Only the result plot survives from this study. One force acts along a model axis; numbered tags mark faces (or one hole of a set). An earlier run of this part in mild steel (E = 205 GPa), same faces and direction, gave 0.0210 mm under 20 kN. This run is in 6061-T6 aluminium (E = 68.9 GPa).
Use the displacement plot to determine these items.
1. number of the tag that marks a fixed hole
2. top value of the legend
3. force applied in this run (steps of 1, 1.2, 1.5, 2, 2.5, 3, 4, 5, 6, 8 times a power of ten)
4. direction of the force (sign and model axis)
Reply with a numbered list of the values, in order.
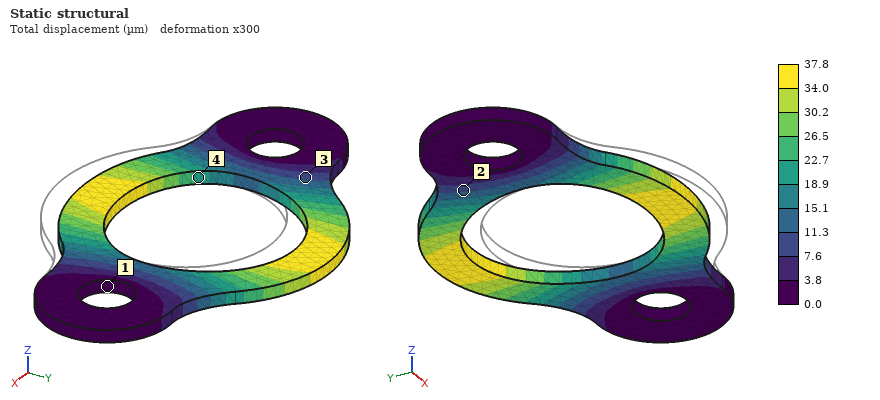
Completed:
1. 1
2. 37.8 µm
3. 12 kN
4. +Y
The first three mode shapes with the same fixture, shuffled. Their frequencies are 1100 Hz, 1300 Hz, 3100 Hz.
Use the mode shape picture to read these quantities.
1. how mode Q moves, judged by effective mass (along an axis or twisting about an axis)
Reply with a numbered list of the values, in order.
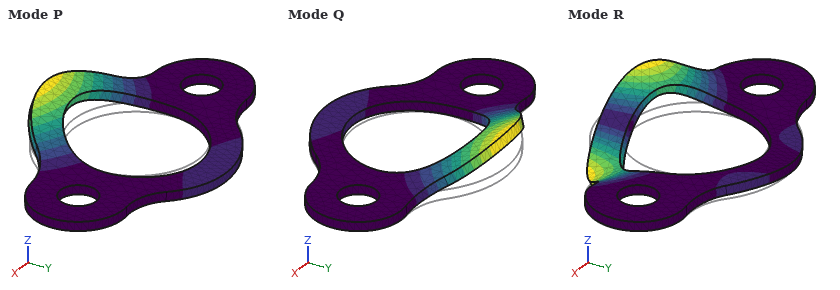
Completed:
1. along Z
